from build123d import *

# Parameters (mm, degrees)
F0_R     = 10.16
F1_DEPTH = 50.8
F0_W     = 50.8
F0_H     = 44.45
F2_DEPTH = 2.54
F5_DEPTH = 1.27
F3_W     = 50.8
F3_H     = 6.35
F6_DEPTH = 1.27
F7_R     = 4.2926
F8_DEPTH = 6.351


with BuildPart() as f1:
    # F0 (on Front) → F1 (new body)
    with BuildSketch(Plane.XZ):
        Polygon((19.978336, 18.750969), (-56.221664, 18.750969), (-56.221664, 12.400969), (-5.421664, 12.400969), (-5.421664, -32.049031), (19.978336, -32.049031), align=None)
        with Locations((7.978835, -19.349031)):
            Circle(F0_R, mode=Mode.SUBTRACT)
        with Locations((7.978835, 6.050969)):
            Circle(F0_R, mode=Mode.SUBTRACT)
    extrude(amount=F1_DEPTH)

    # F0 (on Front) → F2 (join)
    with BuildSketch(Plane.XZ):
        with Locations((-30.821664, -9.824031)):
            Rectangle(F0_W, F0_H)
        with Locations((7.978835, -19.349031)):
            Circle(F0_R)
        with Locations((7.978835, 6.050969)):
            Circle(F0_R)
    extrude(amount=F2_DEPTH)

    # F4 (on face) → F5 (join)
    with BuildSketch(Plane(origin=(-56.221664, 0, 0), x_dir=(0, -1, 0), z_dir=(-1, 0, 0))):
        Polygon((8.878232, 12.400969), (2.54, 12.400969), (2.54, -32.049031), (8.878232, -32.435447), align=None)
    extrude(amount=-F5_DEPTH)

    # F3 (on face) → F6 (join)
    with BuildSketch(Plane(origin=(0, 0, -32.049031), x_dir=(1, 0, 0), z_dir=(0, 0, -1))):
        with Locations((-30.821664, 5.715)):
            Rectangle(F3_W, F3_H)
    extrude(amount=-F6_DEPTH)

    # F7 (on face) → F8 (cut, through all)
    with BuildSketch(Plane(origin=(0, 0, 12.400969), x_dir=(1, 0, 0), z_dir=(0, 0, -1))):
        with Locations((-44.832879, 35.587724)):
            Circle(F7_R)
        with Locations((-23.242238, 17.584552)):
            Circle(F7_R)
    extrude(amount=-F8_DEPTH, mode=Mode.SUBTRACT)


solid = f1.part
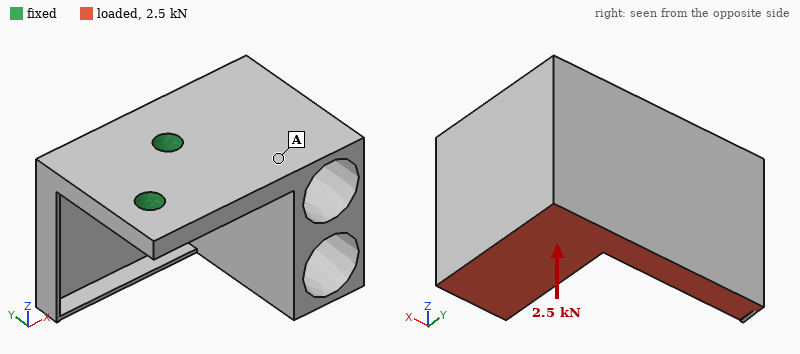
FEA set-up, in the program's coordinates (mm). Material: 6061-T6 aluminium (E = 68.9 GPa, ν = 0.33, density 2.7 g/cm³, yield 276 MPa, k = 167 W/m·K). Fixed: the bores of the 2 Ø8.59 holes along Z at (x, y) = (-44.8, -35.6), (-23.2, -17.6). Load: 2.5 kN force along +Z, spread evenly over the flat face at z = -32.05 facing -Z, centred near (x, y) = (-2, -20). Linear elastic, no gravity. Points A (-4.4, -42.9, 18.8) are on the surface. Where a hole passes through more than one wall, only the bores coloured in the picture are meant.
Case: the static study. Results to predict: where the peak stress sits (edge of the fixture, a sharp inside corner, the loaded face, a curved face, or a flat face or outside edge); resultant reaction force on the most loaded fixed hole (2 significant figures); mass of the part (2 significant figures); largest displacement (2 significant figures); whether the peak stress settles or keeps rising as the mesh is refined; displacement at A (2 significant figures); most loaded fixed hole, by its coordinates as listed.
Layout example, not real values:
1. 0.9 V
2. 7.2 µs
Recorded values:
1. edge of the fixture
2. 2.9 kN
3. 150 g
4. 0.25 mm
5. keeps rising
6. 0.087 mm
7. (-23.2, -17.6)
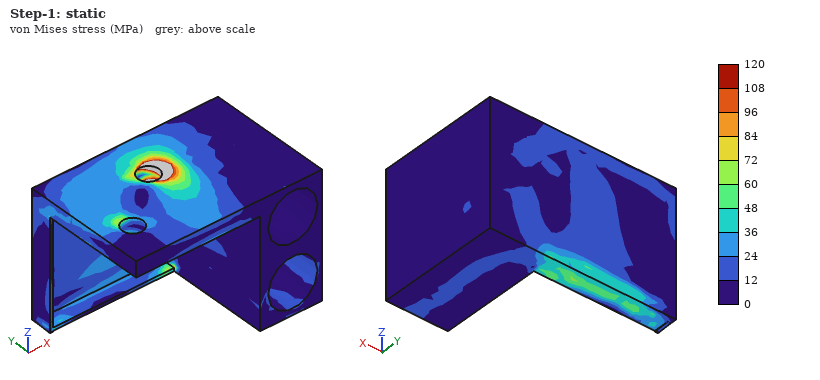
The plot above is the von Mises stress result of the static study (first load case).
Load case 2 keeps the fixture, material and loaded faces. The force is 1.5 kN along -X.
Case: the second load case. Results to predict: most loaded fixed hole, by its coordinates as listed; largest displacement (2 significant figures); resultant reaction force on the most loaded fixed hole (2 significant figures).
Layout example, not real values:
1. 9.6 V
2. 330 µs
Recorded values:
1. (-23.2, -17.6)
2. 0.50 mm
3. 1.4 kN
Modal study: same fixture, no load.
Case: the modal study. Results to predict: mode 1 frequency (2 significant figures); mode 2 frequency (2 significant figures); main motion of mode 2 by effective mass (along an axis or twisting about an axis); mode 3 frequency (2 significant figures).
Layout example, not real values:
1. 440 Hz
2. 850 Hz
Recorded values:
1. 1300 Hz
2. 1600 Hz
3. along Y
4. 2800 Hz
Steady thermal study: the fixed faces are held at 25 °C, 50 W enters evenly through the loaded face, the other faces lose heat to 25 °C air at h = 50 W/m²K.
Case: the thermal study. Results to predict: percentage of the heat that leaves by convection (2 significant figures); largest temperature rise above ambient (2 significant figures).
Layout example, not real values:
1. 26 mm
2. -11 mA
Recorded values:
1. 39 %
2. 31 K
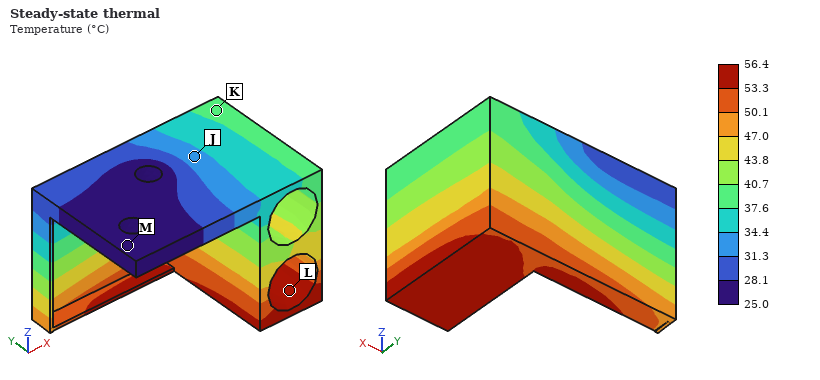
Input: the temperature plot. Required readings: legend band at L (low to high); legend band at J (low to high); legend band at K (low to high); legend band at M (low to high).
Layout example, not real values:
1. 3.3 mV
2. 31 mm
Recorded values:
1. 53.3 to 56.4 °C
2. 31.3 to 34.4 °C
3. 37.6 to 40.7 °C
4. 25.0 to 28.1 °C
